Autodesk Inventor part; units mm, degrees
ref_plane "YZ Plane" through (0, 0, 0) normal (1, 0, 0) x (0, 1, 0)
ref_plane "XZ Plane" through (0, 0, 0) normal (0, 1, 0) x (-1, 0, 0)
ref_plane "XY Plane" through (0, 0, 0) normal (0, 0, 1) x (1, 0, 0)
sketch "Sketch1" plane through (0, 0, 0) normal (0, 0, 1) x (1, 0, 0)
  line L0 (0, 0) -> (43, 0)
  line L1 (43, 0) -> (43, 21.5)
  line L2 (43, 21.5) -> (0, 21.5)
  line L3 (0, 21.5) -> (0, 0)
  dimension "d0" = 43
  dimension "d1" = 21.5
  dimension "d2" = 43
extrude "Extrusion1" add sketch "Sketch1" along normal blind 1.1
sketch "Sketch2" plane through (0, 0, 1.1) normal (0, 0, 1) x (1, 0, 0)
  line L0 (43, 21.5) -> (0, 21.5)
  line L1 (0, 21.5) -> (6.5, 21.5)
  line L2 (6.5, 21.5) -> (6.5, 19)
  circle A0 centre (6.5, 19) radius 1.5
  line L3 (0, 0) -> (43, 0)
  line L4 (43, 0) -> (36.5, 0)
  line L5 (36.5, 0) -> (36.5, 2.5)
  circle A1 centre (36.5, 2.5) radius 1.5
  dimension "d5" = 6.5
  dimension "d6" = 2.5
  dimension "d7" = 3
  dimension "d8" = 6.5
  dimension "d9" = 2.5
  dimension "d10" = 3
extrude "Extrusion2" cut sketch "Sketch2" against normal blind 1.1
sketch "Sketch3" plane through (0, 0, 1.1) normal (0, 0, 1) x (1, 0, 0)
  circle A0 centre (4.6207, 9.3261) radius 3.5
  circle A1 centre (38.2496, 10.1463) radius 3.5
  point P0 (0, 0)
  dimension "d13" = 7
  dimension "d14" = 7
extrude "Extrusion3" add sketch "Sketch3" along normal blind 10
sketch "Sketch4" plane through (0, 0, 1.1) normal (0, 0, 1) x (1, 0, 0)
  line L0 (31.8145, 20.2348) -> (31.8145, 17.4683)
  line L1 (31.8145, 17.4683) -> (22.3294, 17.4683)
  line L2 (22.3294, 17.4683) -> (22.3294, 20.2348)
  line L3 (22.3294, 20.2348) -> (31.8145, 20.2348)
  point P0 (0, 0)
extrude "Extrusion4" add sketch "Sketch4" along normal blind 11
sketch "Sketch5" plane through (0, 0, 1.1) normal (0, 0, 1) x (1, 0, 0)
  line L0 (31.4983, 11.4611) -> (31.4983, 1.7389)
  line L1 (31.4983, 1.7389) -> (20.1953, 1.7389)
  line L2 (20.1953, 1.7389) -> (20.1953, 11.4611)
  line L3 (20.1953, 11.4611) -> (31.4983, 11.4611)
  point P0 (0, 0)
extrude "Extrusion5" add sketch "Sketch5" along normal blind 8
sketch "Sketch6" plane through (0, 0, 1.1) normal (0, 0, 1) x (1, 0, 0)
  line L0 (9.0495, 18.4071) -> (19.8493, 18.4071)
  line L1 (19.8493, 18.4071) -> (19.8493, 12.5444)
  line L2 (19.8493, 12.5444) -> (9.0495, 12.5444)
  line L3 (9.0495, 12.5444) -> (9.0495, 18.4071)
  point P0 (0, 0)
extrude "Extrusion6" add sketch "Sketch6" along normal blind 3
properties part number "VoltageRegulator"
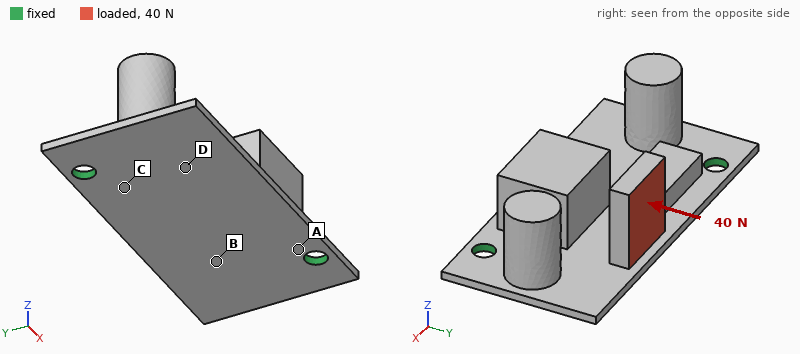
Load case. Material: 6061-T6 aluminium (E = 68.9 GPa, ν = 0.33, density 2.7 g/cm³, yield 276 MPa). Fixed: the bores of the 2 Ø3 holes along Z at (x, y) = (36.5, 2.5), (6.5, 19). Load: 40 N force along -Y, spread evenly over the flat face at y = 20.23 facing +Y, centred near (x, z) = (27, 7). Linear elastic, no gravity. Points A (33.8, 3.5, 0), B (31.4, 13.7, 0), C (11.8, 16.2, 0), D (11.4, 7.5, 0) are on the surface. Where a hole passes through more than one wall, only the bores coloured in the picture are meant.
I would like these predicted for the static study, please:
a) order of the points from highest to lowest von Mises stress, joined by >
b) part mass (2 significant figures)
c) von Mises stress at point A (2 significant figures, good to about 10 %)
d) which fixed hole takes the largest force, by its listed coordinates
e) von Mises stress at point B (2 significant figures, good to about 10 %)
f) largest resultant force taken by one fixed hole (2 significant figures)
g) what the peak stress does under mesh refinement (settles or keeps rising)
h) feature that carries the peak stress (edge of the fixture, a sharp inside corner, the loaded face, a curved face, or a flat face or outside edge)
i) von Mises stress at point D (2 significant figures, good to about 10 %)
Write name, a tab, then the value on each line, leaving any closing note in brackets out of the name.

order of the points from highest to lowest von Mises stress, joined by >	B > A > C > D
part mass	8.4 g
von Mises stress at point A	18 MPa
which fixed hole takes the largest force, by its listed coordinates	(36.5, 2.5)
von Mises stress at point B	23 MPa
largest resultant force taken by one fixed hole	25 N
what the peak stress does under mesh refinement	keeps rising
feature that carries the peak stress	edge of the fixture
von Mises stress at point D	4.7 MPa
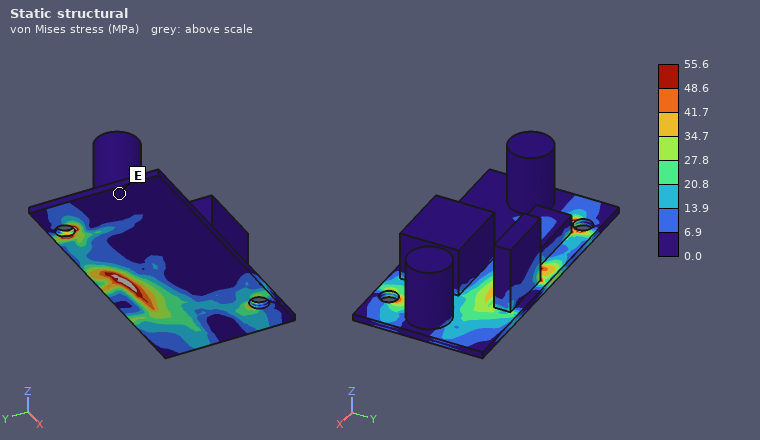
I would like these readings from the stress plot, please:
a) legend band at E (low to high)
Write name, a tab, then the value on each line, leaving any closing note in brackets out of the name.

legend band at E	0.0 to 6.9 MPa
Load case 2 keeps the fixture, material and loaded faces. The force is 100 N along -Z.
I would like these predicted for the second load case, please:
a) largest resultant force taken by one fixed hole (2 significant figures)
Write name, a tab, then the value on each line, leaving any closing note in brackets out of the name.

largest resultant force taken by one fixed hole	65 N
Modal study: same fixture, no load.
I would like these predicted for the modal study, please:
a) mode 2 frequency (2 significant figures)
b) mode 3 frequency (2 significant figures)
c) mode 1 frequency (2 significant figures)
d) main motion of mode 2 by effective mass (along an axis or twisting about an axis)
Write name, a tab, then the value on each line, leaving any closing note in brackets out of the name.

mode 2 frequency	2700 Hz
mode 3 frequency	3400 Hz
mode 1 frequency	2000 Hz
main motion of mode 2 by effective mass	along Z
